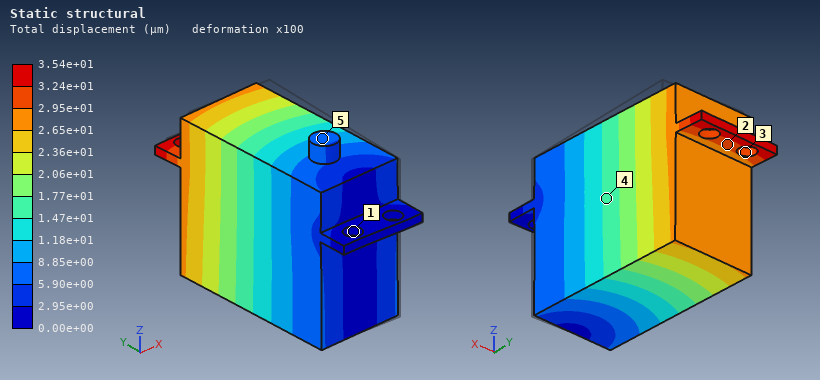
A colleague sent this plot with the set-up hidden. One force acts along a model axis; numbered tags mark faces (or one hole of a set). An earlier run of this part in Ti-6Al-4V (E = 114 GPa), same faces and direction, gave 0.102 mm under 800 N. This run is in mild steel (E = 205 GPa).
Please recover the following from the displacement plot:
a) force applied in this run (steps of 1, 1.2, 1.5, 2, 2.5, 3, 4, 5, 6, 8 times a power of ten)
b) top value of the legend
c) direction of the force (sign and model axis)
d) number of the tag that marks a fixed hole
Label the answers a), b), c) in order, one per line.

a) 500 N
b) 3.54e+01 µm
c) -X
d) 1
